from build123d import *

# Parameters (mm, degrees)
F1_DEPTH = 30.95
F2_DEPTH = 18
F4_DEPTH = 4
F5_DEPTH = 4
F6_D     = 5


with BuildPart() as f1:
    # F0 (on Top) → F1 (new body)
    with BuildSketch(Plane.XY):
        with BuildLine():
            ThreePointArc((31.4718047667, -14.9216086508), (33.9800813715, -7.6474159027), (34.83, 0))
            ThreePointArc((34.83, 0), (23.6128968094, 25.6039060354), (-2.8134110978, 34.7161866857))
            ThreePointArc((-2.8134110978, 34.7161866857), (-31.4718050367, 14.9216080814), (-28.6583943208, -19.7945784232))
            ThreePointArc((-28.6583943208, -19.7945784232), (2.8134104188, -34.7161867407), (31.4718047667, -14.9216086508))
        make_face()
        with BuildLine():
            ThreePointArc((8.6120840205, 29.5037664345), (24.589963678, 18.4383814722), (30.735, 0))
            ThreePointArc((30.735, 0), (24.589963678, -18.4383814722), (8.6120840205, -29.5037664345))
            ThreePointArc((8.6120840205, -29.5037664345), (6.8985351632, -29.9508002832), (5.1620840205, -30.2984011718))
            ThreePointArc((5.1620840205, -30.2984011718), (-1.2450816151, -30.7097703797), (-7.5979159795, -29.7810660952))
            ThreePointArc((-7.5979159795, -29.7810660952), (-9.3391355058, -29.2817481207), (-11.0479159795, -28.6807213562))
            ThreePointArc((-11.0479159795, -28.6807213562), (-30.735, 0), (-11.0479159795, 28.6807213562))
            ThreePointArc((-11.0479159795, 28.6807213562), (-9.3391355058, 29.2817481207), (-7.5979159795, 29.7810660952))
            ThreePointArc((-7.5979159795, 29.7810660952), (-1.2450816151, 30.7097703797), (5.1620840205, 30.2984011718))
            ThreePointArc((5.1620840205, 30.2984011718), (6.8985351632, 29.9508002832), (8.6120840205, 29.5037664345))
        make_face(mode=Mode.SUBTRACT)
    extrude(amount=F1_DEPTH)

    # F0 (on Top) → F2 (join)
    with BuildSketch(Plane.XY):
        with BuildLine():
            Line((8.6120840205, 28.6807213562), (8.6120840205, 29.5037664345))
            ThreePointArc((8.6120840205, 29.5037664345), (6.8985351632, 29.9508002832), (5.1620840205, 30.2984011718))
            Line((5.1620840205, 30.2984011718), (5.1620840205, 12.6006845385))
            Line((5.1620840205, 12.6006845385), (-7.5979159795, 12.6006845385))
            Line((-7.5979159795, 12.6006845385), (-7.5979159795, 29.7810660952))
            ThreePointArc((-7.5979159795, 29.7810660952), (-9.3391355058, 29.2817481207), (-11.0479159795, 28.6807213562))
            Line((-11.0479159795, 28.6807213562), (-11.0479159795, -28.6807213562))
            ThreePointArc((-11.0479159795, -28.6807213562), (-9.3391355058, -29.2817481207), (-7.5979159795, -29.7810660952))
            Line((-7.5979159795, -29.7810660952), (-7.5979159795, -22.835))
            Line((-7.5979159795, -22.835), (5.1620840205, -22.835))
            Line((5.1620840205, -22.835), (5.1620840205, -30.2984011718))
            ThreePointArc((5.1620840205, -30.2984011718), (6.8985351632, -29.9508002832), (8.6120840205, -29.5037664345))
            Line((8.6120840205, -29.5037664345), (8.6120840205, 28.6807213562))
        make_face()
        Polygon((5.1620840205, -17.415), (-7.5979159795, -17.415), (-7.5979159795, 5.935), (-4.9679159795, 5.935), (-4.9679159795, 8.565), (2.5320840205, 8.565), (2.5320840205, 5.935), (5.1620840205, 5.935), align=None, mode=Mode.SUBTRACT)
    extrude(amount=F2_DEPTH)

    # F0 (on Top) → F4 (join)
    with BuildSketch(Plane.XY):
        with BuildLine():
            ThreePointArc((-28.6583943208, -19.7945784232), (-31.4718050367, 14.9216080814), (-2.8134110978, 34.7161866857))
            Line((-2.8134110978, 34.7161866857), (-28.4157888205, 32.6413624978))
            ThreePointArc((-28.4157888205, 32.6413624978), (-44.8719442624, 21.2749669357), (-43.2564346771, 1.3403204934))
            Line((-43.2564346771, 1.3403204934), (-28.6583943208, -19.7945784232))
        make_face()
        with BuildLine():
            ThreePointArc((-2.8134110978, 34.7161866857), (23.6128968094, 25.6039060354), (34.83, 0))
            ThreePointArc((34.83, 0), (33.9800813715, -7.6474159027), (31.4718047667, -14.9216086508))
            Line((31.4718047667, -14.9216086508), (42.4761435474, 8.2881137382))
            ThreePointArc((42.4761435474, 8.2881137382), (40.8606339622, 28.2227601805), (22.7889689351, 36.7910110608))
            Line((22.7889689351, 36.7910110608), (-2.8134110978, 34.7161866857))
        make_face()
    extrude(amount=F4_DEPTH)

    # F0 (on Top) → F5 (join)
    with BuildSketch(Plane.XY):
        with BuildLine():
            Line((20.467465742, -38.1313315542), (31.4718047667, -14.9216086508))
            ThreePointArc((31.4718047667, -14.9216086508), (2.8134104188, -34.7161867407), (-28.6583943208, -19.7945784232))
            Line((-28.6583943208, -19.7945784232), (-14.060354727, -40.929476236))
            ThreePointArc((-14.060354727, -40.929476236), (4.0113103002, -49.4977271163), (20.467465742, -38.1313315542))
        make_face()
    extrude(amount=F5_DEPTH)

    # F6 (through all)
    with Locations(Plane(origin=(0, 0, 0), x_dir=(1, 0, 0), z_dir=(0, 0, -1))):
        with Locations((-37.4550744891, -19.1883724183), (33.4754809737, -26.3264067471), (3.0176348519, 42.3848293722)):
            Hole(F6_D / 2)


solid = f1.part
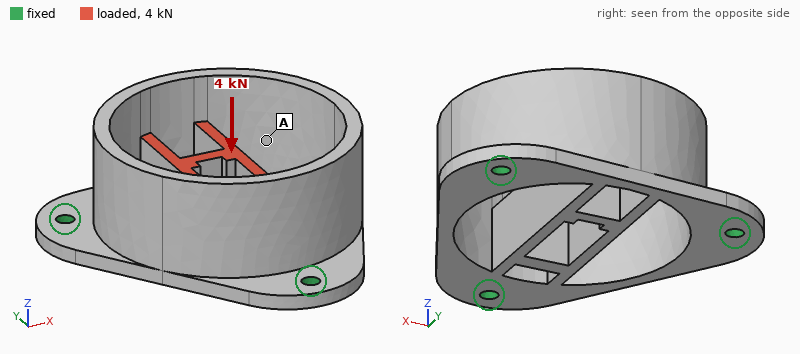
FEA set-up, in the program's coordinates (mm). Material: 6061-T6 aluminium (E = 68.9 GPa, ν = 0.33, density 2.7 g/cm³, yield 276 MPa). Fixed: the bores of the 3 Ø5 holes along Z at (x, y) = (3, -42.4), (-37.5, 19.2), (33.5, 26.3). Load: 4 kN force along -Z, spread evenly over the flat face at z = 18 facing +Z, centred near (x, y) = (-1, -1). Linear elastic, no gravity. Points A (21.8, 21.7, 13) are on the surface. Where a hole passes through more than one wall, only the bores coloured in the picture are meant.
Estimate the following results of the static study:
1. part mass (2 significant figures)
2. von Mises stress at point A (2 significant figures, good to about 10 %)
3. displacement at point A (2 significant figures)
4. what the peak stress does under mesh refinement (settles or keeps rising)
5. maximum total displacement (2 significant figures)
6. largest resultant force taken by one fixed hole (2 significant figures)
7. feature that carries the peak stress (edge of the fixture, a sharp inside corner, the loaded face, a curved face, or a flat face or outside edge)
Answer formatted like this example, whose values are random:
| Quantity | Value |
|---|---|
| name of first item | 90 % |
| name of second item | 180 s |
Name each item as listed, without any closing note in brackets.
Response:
| Quantity | Value |
|---|---|
| part mass | 110 g |
| von Mises stress at point A | 18 MPa |
| displacement at point A | 29 µm |
| what the peak stress does under mesh refinement | keeps rising |
| maximum total displacement | 73 µm |
| largest resultant force taken by one fixed hole | 1.6 kN |
| feature that carries the peak stress | edge of the fixture |
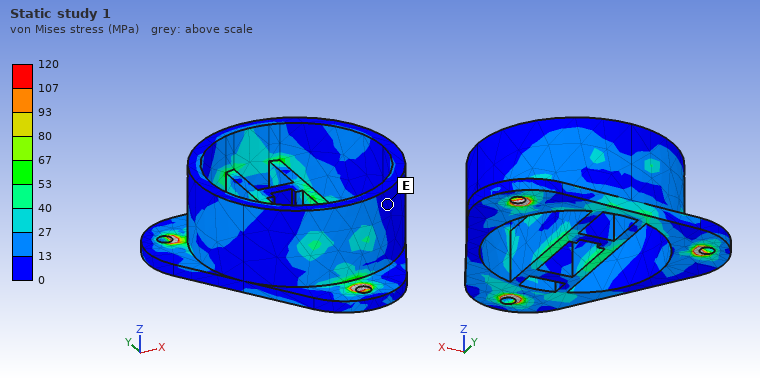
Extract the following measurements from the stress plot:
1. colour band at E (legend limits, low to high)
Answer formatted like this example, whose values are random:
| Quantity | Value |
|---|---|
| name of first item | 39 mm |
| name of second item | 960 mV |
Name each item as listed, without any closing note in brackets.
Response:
| Quantity | Value |
|---|---|
| colour band at E | 0 to 13 MPa |
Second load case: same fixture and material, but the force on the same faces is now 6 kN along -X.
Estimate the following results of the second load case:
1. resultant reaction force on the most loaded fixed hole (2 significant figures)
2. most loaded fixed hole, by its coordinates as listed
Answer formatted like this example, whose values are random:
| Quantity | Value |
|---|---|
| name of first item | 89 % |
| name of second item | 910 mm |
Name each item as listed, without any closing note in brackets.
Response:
| Quantity | Value |
|---|---|
| resultant reaction force on the most loaded fixed hole | 2.7 kN |
| most loaded fixed hole, by its coordinates as listed | (3, -42.4) |
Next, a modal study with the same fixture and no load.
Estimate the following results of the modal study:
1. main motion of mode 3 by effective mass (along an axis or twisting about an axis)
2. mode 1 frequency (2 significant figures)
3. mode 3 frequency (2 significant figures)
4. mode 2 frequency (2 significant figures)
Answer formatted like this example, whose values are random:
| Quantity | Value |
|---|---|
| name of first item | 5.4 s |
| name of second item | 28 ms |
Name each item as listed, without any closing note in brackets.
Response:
| Quantity | Value |
|---|---|
| main motion of mode 3 by effective mass | along Z |
| mode 1 frequency | 3600 Hz |
| mode 3 frequency | 5300 Hz |
| mode 2 frequency | 5100 Hz |
